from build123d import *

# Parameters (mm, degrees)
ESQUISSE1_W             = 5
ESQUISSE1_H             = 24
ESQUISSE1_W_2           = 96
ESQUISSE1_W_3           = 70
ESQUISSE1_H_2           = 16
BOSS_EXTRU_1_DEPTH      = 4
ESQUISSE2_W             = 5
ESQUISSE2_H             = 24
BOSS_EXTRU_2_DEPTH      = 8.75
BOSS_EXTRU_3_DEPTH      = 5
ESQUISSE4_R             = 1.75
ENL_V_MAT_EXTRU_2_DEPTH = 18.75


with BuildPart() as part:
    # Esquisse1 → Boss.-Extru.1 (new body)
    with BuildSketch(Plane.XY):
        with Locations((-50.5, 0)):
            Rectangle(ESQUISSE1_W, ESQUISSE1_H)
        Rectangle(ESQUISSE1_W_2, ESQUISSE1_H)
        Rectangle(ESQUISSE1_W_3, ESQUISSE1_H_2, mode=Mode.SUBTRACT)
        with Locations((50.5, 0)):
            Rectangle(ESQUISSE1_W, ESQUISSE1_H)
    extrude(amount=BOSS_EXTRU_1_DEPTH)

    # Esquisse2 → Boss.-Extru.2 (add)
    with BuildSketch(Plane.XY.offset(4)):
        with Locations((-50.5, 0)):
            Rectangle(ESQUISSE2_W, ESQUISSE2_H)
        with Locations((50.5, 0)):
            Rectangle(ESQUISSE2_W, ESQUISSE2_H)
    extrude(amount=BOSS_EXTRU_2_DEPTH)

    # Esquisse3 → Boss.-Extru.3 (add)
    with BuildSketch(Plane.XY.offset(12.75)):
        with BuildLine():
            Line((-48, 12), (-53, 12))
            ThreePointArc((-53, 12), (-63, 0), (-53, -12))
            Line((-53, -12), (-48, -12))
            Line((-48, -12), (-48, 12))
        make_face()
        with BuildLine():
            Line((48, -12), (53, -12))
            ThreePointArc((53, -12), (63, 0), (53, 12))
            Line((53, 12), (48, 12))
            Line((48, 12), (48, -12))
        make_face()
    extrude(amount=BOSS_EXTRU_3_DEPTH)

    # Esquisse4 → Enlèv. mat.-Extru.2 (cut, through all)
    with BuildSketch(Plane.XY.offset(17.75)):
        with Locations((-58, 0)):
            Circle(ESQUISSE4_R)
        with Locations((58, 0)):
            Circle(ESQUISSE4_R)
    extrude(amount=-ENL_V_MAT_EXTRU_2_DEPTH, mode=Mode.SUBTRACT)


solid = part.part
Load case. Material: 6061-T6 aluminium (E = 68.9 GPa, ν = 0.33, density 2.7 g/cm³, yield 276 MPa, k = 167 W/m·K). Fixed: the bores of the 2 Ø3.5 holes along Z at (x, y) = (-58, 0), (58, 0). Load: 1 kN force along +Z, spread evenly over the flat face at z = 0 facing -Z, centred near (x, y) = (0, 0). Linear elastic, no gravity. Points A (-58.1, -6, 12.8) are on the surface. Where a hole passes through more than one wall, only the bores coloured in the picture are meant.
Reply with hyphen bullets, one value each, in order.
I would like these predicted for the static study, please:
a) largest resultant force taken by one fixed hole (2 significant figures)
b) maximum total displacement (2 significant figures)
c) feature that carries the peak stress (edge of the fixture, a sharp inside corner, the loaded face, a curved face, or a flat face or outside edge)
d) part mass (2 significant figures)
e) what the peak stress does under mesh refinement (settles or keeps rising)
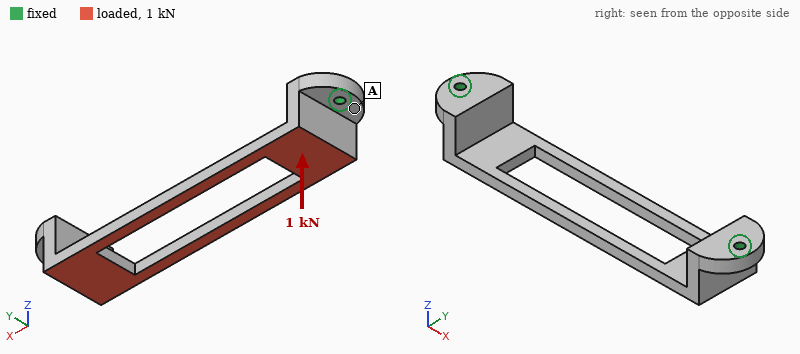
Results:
- 790 N
- 0.37 mm
- edge of the fixture
- 29 g
- keeps rising
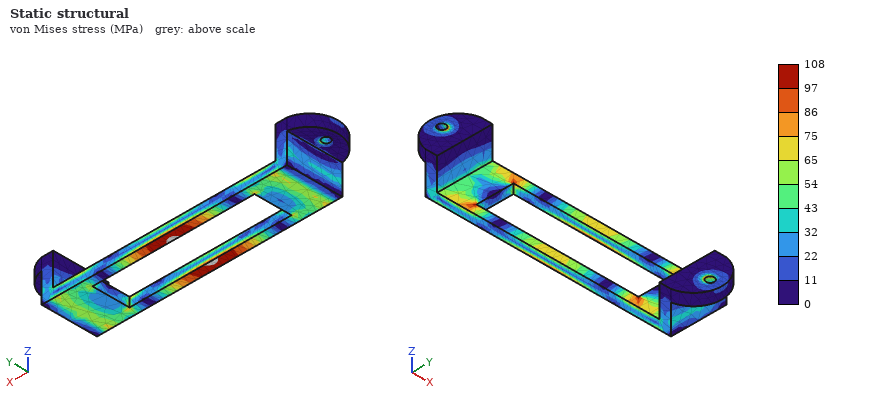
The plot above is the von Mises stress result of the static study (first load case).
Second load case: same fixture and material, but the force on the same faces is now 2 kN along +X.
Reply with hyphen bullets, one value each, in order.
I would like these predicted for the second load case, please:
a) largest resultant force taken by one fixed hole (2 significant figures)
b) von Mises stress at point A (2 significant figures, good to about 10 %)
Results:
- 1.0 kN
- 78 MPa
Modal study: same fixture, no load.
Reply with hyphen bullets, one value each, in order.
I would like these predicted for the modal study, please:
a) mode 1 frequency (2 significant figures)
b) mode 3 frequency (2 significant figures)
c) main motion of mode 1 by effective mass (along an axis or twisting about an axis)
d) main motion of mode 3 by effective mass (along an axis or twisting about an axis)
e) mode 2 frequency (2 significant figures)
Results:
- 2500 Hz
- 3300 Hz
- along Z
- along Y
- 2900 Hz
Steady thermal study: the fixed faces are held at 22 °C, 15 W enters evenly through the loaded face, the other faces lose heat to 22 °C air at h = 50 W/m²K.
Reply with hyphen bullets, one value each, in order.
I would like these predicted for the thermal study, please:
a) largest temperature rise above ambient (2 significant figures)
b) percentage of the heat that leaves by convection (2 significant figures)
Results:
- 18 K
- 15 %
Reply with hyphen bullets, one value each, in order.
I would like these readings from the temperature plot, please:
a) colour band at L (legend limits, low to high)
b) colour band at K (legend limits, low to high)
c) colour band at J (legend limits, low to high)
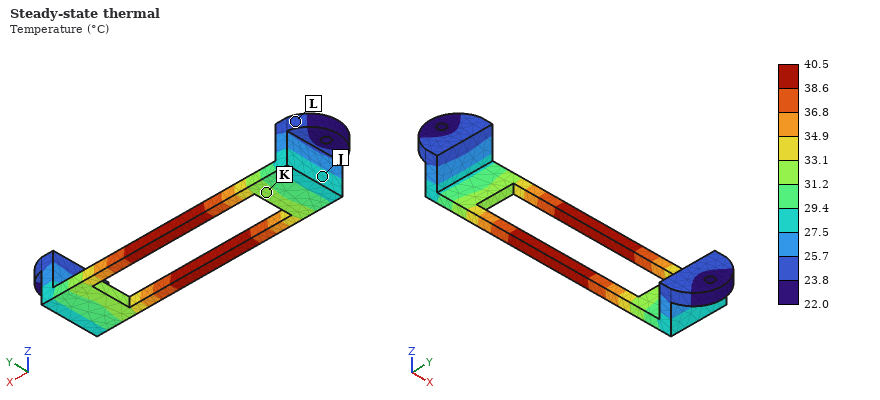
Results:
- 23.8 to 25.7 °C
- 31.2 to 33.1 °C
- 27.5 to 29.4 °C
